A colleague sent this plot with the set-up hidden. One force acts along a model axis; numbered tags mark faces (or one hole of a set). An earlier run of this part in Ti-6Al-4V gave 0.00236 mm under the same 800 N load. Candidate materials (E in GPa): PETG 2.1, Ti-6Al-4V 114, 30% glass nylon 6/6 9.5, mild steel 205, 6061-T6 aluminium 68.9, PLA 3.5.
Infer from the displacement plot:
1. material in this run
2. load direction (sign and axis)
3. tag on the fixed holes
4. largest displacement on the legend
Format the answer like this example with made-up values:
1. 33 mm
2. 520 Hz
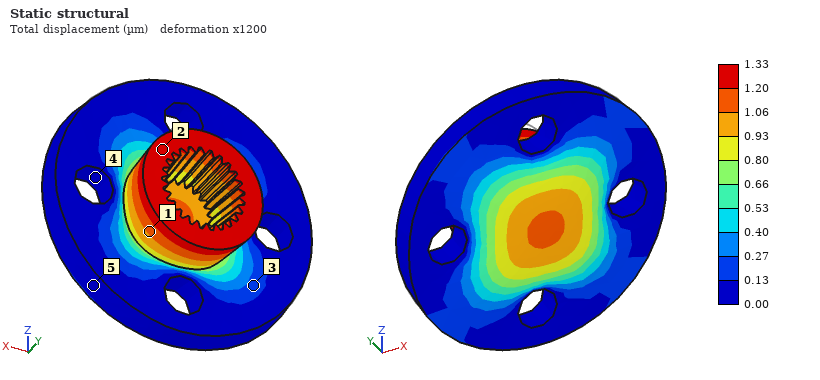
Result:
1. mild steel
2. -Y
3. 4
4. 1.33 µm
